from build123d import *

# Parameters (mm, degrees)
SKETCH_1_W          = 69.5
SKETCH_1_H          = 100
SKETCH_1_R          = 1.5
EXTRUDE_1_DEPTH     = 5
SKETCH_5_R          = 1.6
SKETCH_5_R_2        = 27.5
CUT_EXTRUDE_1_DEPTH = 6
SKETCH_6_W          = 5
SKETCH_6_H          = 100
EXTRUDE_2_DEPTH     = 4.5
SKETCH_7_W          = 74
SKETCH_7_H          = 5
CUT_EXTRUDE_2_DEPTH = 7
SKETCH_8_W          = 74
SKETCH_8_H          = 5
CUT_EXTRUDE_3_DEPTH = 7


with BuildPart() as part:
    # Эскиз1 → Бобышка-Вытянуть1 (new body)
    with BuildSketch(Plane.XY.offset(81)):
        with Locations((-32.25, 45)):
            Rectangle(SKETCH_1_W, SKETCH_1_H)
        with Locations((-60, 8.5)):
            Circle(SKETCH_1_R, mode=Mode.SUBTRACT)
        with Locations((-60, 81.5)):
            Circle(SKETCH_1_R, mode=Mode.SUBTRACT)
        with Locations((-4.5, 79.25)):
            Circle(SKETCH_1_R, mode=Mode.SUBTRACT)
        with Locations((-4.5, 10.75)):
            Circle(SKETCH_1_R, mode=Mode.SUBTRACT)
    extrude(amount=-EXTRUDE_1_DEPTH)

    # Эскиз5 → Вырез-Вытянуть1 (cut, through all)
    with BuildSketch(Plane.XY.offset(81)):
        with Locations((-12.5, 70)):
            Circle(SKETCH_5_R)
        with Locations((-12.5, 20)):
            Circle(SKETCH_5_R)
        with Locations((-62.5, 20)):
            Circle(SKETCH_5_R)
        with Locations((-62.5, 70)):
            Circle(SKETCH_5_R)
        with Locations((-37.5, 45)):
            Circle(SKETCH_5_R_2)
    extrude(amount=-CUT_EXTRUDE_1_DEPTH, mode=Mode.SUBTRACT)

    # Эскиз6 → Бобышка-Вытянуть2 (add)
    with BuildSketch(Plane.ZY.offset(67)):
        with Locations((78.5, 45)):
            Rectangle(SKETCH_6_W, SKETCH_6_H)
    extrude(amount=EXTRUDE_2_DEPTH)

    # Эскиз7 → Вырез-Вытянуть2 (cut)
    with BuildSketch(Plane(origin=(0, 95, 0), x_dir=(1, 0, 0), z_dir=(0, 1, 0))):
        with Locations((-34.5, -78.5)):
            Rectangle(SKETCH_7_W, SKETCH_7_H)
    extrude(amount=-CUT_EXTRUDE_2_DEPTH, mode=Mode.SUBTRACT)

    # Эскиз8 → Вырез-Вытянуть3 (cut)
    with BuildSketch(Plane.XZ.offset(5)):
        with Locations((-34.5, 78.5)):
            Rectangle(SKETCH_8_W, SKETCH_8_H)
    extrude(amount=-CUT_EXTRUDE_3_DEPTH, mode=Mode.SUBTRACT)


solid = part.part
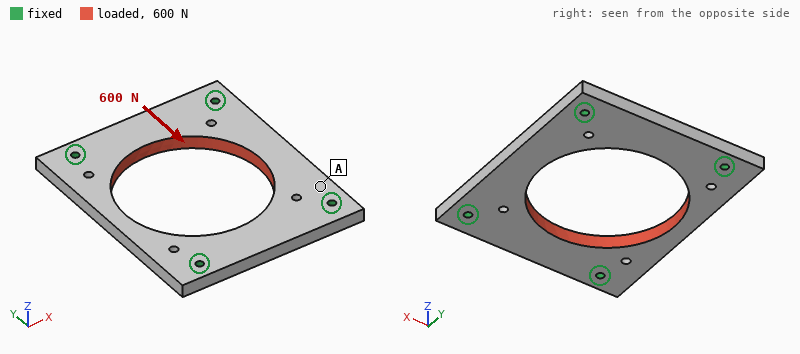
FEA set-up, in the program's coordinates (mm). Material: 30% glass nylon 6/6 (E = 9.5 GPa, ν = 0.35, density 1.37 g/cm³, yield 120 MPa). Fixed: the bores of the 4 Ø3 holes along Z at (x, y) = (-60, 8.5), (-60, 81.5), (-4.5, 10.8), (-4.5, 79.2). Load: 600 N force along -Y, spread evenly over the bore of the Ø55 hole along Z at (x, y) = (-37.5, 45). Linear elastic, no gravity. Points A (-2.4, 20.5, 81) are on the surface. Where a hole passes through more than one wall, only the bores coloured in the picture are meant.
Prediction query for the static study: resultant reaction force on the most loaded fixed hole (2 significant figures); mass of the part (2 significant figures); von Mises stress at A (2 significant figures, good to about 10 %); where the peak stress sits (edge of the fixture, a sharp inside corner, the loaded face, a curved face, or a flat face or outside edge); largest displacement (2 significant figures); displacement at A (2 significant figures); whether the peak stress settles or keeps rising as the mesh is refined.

160 N
27 g
1.6 MPa
edge of the fixture
11 µm
2.1 µm
keeps rising
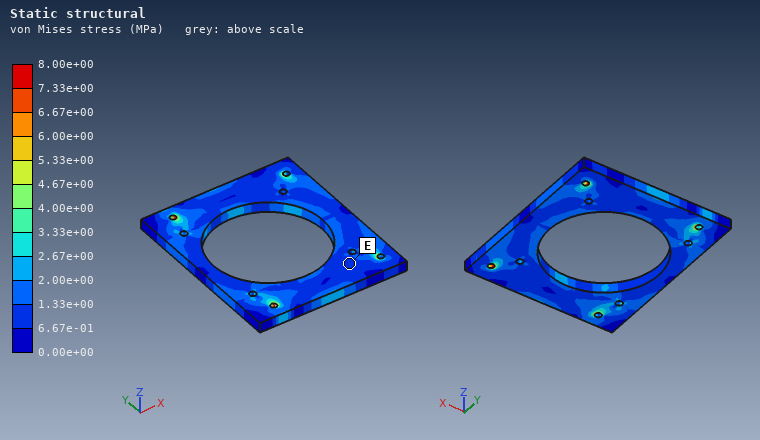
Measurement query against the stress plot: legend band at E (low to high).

6.67e-01 to 1.33e+00 MPa
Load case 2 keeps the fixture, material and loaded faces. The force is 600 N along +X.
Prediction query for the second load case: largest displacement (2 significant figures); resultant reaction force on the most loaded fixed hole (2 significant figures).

31 µm
160 N
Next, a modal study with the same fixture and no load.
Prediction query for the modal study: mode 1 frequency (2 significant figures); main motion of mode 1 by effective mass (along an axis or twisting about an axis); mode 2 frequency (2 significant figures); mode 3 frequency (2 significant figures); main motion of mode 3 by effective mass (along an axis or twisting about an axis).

2800 Hz
along Z
2900 Hz
3900 Hz
along Z
